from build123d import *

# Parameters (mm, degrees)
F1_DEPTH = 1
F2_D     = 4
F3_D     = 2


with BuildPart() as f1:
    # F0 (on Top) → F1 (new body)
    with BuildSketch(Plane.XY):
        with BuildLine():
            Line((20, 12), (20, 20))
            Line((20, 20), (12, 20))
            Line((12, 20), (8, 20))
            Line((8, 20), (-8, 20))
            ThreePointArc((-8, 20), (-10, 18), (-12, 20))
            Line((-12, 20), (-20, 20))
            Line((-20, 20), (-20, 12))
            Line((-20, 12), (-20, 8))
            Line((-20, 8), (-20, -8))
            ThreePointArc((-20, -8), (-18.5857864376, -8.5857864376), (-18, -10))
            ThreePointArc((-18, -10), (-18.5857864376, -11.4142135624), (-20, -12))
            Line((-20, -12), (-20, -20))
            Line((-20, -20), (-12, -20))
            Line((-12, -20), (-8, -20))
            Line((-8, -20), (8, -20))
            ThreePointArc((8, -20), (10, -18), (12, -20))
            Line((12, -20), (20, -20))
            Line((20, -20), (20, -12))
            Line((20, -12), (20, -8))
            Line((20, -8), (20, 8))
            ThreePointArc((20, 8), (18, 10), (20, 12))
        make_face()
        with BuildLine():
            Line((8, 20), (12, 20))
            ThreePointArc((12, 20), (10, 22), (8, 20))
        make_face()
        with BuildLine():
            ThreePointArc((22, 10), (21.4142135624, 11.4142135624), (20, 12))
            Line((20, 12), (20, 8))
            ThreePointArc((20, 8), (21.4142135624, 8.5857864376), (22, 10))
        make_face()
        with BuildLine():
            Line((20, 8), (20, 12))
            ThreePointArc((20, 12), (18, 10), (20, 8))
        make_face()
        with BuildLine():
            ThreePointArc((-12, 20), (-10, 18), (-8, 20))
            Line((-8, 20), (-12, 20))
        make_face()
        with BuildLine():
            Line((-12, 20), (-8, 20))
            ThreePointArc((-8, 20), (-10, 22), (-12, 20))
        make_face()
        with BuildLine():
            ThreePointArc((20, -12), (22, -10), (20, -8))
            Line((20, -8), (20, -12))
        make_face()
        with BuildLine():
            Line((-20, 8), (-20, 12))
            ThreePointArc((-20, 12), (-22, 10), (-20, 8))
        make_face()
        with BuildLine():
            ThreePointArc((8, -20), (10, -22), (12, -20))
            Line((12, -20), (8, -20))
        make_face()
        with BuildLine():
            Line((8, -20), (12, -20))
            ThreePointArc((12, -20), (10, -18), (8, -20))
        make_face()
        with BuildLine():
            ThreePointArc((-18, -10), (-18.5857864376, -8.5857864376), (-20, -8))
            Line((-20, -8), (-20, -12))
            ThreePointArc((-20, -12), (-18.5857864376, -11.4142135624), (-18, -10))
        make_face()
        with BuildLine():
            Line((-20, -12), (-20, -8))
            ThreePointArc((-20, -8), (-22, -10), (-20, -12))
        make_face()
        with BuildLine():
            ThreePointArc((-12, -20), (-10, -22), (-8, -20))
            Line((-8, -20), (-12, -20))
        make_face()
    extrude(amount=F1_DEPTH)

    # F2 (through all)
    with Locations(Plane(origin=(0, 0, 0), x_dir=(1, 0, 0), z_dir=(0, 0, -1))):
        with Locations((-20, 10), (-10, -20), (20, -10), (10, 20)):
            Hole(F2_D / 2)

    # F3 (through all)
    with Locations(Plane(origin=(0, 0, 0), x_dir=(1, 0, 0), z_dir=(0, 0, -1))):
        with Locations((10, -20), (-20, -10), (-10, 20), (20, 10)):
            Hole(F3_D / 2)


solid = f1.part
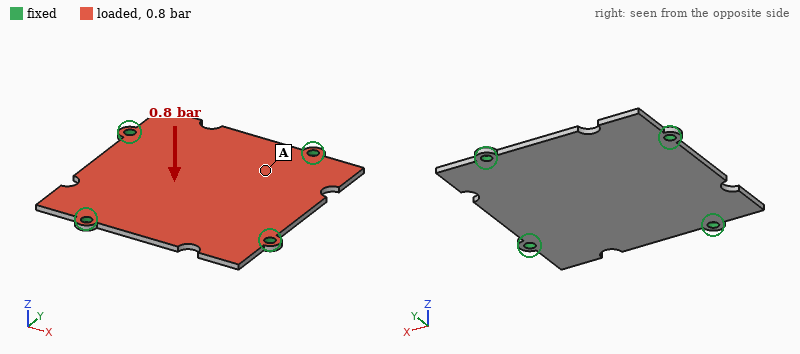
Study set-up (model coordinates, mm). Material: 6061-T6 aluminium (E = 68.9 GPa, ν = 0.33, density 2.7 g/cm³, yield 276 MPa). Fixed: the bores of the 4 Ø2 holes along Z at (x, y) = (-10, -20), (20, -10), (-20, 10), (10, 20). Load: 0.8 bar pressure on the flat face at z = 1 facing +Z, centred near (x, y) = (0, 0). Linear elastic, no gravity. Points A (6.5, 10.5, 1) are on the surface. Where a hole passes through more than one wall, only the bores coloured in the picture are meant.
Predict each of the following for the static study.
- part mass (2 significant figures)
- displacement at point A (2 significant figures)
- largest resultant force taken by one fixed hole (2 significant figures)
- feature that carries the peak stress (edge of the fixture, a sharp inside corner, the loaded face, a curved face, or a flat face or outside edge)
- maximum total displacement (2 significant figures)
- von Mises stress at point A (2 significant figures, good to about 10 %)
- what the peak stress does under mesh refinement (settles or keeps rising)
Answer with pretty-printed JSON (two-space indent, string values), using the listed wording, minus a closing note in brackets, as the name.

{
  "part mass": "4.3 g",
  "displacement at point A": "55 µm",
  "largest resultant force taken by one fixed hole": "32 N",
  "feature that carries the peak stress": "edge of the fixture",
  "maximum total displacement": "92 µm",
  "von Mises stress at point A": "14 MPa",
  "what the peak stress does under mesh refinement": "keeps rising"
}
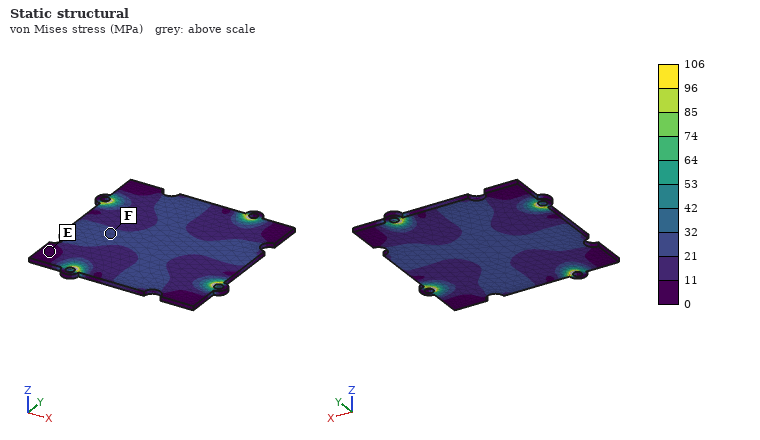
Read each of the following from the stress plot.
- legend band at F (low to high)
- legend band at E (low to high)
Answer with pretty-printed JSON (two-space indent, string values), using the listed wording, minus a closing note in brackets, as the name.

{
  "legend band at F": "21 to 32 MPa",
  "legend band at E": "0 to 11 MPa"
}
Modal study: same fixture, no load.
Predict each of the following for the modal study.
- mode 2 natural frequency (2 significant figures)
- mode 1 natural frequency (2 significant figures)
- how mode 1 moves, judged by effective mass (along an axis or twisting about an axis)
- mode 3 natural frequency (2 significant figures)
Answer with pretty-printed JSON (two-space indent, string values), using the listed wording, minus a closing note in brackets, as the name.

{
  "mode 2 natural frequency": "5000 Hz",
  "mode 1 natural frequency": "3500 Hz",
  "how mode 1 moves, judged by effective mass": "along Z",
  "mode 3 natural frequency": "5100 Hz"
}
